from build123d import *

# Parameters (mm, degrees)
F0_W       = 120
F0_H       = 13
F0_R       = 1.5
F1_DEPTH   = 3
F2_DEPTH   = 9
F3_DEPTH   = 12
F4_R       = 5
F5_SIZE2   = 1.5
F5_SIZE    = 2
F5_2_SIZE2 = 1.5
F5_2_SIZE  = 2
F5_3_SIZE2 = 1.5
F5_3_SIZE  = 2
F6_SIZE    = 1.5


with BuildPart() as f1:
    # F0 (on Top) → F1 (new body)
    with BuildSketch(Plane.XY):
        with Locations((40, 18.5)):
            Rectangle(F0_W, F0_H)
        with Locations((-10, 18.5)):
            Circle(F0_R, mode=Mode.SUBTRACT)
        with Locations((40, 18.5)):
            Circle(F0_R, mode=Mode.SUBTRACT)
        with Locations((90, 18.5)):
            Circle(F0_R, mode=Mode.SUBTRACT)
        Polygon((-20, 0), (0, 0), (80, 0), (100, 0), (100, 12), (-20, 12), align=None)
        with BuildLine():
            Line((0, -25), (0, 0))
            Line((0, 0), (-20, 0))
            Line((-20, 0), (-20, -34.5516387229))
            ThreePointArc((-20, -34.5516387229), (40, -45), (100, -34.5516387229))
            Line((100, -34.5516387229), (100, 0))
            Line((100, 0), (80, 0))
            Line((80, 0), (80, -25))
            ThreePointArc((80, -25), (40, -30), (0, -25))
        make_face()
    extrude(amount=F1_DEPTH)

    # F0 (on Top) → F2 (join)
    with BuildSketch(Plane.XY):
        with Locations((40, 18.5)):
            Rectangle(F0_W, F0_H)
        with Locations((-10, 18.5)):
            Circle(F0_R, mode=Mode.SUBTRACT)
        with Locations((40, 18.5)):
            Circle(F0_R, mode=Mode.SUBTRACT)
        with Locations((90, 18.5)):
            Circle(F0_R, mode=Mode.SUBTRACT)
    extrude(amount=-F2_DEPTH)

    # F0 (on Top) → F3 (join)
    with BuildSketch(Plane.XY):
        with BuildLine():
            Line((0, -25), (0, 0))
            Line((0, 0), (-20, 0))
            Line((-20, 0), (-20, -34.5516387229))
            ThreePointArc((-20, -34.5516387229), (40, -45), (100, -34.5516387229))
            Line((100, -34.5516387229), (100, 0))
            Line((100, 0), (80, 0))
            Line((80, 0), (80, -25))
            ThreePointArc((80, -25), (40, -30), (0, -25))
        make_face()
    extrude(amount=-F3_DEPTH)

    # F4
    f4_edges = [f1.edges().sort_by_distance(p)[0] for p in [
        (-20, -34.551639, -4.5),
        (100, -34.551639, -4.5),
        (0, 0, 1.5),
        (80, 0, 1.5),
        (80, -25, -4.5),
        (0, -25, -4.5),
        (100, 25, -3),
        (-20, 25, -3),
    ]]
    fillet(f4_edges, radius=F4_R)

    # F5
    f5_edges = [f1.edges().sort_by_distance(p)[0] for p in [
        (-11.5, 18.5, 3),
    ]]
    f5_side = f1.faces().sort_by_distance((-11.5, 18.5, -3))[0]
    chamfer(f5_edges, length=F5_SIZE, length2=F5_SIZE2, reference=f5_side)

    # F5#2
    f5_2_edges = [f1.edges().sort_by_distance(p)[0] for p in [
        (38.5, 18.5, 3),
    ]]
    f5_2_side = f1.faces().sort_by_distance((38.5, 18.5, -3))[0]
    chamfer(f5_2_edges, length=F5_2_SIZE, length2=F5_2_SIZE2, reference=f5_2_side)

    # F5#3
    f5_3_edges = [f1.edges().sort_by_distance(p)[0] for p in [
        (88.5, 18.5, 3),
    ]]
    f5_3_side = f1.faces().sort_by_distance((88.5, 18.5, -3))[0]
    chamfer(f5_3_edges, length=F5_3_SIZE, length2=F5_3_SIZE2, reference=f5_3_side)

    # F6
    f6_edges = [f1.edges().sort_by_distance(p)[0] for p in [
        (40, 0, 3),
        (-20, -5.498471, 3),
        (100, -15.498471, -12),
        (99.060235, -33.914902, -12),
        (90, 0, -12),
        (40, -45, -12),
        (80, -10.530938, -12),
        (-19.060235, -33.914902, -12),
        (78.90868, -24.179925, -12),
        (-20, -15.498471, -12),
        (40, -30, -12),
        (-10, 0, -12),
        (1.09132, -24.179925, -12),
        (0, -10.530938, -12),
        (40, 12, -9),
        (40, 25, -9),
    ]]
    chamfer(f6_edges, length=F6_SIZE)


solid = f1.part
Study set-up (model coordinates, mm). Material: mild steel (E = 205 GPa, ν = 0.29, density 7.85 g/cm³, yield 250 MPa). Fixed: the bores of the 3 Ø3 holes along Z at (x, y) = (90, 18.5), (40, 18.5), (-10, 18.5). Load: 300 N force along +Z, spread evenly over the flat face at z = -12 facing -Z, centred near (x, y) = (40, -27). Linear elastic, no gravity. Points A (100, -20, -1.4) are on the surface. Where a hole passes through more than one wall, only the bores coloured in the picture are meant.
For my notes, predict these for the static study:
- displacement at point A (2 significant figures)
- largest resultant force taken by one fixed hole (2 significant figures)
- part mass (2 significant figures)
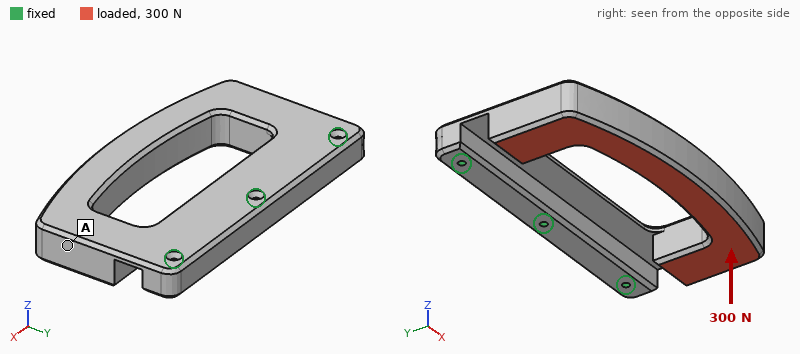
0.15 mm
140 N
490 g
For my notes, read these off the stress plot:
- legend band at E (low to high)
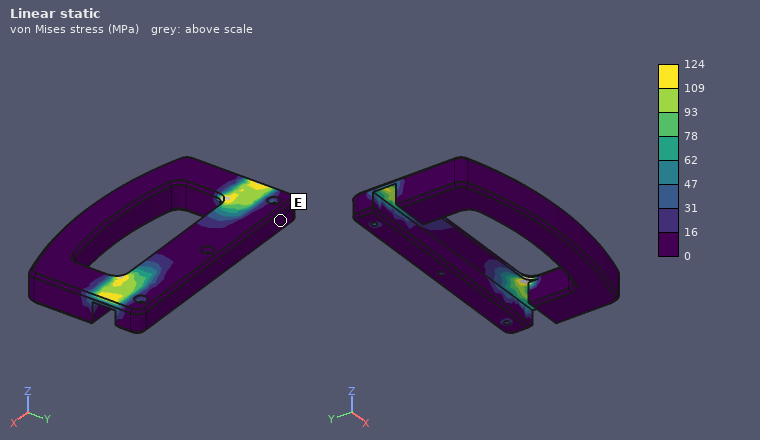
0 to 16 MPa
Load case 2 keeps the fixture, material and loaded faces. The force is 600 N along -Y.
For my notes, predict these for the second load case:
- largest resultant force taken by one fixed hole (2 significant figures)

320 N
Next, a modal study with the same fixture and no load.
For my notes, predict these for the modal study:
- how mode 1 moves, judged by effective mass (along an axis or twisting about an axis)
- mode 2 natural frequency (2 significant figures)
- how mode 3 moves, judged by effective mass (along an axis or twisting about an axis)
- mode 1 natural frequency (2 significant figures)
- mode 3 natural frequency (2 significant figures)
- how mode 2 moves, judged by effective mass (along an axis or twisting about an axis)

along Z
1600 Hz
along X
330 Hz
2900 Hz
twisting about Y
